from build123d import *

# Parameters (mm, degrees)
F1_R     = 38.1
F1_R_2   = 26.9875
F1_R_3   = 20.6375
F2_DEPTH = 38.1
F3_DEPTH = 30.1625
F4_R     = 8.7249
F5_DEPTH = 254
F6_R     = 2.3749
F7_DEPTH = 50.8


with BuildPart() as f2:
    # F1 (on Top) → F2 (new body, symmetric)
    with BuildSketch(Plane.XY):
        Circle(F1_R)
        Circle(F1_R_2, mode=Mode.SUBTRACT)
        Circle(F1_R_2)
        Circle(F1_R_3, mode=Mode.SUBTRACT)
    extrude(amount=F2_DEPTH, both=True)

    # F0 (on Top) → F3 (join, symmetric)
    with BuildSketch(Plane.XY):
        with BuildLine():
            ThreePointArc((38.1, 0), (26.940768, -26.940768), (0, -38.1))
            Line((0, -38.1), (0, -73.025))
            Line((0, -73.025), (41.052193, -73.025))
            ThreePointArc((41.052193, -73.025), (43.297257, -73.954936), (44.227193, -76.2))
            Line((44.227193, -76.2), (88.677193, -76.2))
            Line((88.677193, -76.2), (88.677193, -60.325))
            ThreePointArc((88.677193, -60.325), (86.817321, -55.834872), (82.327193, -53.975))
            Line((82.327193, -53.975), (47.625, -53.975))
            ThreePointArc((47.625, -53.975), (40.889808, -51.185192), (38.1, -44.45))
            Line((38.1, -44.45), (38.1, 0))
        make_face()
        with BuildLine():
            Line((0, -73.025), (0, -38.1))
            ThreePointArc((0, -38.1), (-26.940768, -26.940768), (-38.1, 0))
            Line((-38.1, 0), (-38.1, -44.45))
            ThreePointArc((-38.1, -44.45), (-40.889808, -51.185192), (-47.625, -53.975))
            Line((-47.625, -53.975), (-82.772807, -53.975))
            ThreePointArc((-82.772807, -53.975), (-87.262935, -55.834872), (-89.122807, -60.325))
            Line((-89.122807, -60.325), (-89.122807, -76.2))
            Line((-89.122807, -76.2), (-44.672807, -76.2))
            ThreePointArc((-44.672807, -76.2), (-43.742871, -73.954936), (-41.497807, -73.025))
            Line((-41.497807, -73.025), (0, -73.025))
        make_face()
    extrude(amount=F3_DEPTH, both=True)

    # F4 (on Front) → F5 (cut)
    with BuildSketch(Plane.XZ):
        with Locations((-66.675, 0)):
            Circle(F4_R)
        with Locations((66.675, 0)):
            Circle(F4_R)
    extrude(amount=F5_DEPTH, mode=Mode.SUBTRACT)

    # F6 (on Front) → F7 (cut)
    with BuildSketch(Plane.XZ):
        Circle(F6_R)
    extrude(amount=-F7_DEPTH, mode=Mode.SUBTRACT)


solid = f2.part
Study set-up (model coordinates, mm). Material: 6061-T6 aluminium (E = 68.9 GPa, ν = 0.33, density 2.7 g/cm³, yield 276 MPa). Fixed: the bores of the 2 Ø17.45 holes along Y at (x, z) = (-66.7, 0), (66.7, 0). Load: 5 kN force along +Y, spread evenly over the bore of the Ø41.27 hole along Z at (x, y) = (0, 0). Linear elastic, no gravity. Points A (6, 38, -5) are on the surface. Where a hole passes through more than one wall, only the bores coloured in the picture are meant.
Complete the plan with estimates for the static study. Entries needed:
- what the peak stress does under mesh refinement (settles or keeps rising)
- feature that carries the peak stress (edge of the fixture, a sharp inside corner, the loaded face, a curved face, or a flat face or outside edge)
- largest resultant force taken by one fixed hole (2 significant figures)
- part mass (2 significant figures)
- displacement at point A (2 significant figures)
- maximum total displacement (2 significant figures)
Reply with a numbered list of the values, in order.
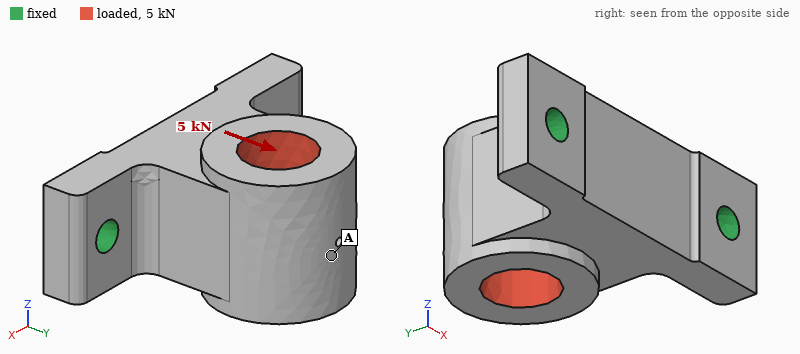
1. keeps rising
2. edge of the fixture
3. 2.8 kN
4. 1.5 kg
5. 7.1 µm
6. 7.3 µm
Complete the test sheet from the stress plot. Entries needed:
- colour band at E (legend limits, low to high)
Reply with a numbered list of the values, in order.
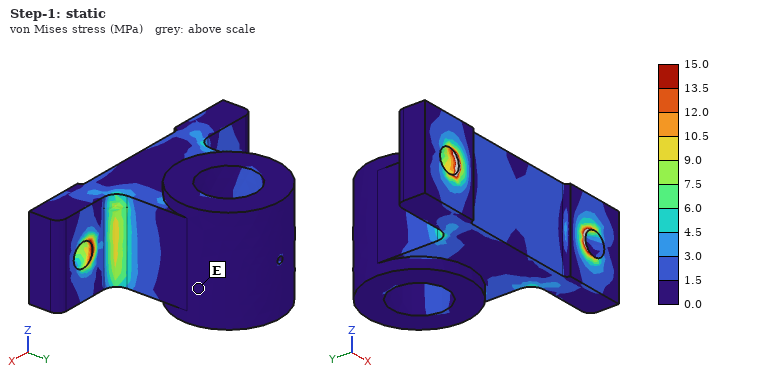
1. 0.0 to 1.5 MPa
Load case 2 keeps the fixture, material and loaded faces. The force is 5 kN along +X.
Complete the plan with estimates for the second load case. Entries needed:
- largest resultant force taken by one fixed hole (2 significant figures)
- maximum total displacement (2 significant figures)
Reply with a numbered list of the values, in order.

1. 4.0 kN
2. 22 µm
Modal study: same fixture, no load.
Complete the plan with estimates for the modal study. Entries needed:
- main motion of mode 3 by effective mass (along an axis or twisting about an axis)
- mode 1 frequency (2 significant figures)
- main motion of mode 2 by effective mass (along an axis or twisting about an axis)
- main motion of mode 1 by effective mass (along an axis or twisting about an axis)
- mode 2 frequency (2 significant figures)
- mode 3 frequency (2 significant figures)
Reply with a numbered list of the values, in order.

1. along Y
2. 1400 Hz
3. along X
4. along Z
5. 3200 Hz
6. 4200 Hz
